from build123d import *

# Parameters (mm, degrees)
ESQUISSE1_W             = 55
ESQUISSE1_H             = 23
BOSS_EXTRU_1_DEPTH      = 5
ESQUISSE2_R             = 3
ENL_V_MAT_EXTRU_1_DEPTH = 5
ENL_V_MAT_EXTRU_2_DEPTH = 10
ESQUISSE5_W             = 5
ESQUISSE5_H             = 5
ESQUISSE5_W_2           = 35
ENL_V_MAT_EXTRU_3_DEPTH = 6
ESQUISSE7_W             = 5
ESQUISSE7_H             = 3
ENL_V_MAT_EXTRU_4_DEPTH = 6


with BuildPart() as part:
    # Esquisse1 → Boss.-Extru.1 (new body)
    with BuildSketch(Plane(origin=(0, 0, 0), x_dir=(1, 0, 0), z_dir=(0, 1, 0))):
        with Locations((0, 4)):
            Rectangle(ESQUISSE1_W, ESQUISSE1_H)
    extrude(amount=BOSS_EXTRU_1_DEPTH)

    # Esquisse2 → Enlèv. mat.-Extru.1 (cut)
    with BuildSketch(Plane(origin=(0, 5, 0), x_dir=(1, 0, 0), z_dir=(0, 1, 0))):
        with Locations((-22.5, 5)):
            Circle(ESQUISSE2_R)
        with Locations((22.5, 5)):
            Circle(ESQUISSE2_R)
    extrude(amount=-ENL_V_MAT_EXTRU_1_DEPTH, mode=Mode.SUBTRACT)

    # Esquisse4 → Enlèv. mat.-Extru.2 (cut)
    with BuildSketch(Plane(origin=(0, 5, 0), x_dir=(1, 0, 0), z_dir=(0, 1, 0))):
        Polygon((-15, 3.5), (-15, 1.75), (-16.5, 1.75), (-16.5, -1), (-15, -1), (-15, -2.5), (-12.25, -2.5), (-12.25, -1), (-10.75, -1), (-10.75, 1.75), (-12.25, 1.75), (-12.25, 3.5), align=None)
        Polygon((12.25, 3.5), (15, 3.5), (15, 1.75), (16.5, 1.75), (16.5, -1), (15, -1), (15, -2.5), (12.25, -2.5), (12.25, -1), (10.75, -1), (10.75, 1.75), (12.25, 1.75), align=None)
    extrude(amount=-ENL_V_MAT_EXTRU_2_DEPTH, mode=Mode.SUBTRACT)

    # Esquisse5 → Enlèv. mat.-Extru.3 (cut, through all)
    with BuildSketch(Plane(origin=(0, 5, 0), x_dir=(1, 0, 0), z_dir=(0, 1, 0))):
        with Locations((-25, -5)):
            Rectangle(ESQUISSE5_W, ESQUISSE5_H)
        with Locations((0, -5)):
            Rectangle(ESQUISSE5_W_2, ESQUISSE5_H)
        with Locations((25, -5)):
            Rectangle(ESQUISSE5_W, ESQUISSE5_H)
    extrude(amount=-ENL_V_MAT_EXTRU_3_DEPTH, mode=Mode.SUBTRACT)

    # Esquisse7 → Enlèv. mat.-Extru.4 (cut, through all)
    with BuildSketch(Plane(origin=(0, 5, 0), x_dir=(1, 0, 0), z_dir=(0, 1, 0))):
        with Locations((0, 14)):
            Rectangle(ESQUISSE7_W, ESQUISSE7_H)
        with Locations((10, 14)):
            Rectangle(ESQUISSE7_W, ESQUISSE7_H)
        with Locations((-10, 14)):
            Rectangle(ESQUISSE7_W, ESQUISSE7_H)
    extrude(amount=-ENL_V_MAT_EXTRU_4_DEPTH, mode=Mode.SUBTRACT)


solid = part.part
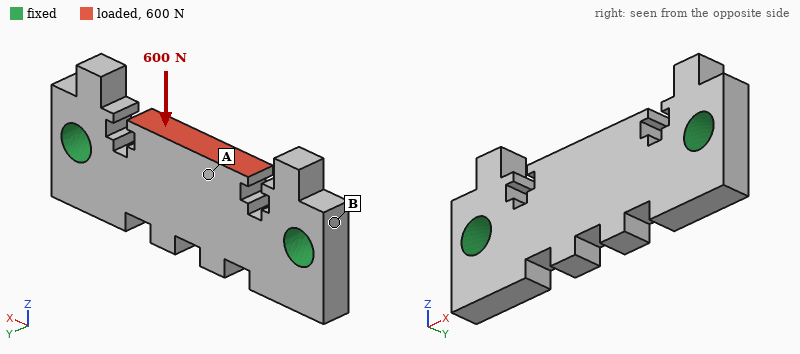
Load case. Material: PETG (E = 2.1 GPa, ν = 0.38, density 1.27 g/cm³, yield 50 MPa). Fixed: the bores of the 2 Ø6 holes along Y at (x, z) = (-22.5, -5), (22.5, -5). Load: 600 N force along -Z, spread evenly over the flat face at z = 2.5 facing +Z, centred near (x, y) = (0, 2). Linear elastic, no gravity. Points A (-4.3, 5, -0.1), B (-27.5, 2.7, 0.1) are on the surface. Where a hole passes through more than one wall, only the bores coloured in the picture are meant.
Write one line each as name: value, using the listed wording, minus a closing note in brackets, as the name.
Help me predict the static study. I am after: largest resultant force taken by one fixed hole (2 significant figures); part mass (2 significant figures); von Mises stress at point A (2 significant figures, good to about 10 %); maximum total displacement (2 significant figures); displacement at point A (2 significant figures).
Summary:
largest resultant force taken by one fixed hole: 300 N
part mass: 5.6 g
von Mises stress at point A: 6.9 MPa
maximum total displacement: 0.23 mm
displacement at point A: 0.21 mm
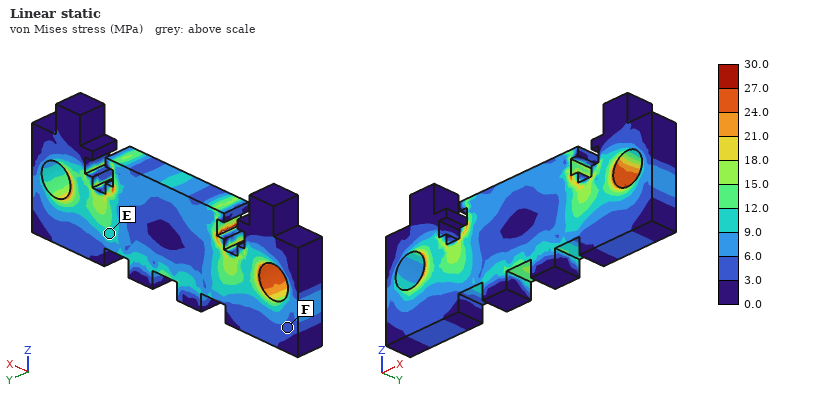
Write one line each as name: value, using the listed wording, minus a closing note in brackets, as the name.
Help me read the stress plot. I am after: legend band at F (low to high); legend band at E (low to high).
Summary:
legend band at F: 3.0 to 6.0 MPa
legend band at E: 9.0 to 12.0 MPa
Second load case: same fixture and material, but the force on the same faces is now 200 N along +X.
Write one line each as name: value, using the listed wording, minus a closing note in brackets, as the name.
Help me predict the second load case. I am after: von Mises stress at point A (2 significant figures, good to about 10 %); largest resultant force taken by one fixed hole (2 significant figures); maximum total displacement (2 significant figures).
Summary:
von Mises stress at point A: 3.8 MPa
largest resultant force taken by one fixed hole: 120 N
maximum total displacement: 86 µm
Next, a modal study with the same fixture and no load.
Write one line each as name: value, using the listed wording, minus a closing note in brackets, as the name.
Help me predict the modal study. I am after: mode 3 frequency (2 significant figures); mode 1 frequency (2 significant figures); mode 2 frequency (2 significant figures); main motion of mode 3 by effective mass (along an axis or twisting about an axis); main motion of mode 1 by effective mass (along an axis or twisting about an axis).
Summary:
mode 3 frequency: 5200 Hz
mode 1 frequency: 3000 Hz
mode 2 frequency: 4000 Hz
main motion of mode 3 by effective mass: along Z
main motion of mode 1 by effective mass: along Y
